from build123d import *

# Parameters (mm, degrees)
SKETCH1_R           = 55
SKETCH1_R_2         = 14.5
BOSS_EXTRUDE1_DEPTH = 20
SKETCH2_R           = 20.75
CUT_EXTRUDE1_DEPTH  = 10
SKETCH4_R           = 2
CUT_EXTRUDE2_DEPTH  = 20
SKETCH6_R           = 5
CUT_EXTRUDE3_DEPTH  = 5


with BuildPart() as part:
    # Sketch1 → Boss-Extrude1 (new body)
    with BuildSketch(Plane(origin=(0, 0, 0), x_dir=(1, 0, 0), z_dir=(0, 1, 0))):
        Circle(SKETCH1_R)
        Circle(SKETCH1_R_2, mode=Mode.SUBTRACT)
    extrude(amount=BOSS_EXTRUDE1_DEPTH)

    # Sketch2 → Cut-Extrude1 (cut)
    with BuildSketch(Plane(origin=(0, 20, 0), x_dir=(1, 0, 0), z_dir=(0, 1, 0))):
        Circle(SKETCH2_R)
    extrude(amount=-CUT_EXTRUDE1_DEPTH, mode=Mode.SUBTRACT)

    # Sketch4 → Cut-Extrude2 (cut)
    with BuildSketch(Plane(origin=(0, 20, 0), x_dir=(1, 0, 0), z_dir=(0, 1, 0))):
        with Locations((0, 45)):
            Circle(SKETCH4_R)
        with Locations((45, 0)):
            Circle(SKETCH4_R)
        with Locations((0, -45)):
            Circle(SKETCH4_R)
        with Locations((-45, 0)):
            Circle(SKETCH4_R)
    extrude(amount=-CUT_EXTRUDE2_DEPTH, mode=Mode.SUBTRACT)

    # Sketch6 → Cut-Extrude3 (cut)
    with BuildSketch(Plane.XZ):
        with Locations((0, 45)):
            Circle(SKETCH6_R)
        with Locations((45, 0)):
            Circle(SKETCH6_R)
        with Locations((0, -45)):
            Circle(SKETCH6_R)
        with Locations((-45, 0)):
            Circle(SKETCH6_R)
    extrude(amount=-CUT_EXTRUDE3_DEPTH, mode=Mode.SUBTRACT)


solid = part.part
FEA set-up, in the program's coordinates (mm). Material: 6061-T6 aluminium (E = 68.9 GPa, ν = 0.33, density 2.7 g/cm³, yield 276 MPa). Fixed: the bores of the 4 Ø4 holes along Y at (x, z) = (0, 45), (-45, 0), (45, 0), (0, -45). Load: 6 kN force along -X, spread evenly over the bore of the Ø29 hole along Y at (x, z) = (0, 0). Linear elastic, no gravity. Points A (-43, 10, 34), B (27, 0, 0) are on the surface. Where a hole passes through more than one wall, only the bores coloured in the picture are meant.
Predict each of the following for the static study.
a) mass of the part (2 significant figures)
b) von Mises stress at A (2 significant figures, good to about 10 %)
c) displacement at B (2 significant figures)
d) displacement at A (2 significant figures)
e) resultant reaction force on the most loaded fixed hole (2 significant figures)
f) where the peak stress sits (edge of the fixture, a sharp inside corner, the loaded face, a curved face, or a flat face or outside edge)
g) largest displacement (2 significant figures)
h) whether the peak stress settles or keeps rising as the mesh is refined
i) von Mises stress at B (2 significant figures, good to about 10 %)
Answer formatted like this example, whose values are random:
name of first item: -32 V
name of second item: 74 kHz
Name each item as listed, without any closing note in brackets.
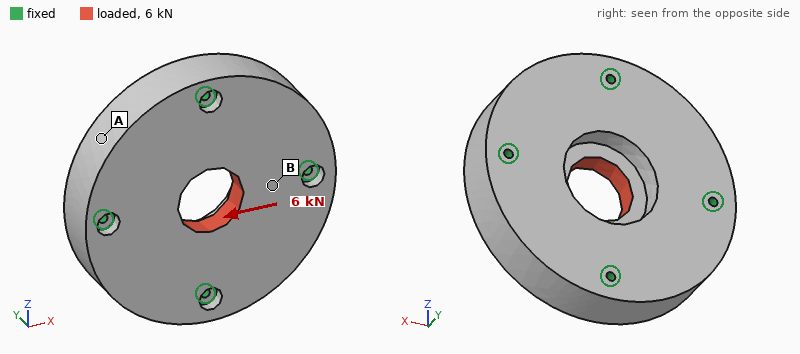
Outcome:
mass of the part: 450 g
von Mises stress at A: 1.6 MPa
displacement at B: 2.4 µm
displacement at A: 1.8 µm
resultant reaction force on the most loaded fixed hole: 1.8 kN
where the peak stress sits: edge of the fixture
largest displacement: 3.9 µm
whether the peak stress settles or keeps rising as the mesh is refined: keeps rising
von Mises stress at B: 7.2 MPa
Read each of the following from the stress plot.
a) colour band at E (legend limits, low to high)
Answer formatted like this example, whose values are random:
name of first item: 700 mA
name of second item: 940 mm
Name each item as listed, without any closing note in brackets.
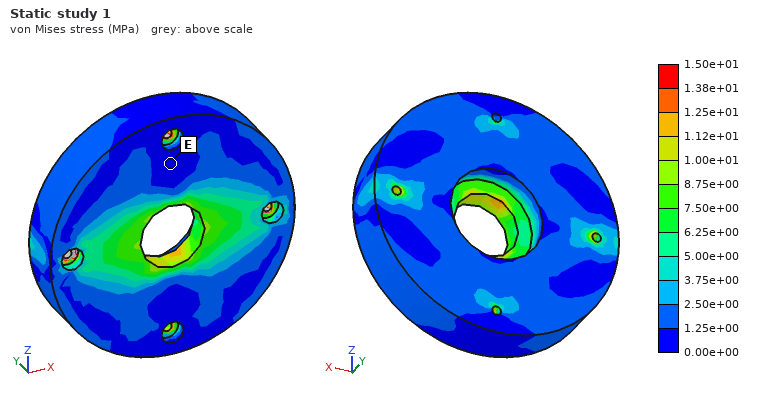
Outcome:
colour band at E: 0.00e+00 to 1.25e+00 MPa
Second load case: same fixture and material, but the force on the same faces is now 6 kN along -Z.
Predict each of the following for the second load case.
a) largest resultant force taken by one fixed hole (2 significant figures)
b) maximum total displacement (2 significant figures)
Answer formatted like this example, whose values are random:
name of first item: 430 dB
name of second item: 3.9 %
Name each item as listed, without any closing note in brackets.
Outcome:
largest resultant force taken by one fixed hole: 1.8 kN
maximum total displacement: 3.9 µm
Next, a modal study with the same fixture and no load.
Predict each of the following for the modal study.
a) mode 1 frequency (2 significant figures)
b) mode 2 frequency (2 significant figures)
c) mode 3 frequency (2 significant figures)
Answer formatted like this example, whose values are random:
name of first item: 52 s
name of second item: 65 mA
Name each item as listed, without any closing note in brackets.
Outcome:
mode 1 frequency: 9800 Hz
mode 2 frequency: 11 kHz
mode 3 frequency: 11 kHz
